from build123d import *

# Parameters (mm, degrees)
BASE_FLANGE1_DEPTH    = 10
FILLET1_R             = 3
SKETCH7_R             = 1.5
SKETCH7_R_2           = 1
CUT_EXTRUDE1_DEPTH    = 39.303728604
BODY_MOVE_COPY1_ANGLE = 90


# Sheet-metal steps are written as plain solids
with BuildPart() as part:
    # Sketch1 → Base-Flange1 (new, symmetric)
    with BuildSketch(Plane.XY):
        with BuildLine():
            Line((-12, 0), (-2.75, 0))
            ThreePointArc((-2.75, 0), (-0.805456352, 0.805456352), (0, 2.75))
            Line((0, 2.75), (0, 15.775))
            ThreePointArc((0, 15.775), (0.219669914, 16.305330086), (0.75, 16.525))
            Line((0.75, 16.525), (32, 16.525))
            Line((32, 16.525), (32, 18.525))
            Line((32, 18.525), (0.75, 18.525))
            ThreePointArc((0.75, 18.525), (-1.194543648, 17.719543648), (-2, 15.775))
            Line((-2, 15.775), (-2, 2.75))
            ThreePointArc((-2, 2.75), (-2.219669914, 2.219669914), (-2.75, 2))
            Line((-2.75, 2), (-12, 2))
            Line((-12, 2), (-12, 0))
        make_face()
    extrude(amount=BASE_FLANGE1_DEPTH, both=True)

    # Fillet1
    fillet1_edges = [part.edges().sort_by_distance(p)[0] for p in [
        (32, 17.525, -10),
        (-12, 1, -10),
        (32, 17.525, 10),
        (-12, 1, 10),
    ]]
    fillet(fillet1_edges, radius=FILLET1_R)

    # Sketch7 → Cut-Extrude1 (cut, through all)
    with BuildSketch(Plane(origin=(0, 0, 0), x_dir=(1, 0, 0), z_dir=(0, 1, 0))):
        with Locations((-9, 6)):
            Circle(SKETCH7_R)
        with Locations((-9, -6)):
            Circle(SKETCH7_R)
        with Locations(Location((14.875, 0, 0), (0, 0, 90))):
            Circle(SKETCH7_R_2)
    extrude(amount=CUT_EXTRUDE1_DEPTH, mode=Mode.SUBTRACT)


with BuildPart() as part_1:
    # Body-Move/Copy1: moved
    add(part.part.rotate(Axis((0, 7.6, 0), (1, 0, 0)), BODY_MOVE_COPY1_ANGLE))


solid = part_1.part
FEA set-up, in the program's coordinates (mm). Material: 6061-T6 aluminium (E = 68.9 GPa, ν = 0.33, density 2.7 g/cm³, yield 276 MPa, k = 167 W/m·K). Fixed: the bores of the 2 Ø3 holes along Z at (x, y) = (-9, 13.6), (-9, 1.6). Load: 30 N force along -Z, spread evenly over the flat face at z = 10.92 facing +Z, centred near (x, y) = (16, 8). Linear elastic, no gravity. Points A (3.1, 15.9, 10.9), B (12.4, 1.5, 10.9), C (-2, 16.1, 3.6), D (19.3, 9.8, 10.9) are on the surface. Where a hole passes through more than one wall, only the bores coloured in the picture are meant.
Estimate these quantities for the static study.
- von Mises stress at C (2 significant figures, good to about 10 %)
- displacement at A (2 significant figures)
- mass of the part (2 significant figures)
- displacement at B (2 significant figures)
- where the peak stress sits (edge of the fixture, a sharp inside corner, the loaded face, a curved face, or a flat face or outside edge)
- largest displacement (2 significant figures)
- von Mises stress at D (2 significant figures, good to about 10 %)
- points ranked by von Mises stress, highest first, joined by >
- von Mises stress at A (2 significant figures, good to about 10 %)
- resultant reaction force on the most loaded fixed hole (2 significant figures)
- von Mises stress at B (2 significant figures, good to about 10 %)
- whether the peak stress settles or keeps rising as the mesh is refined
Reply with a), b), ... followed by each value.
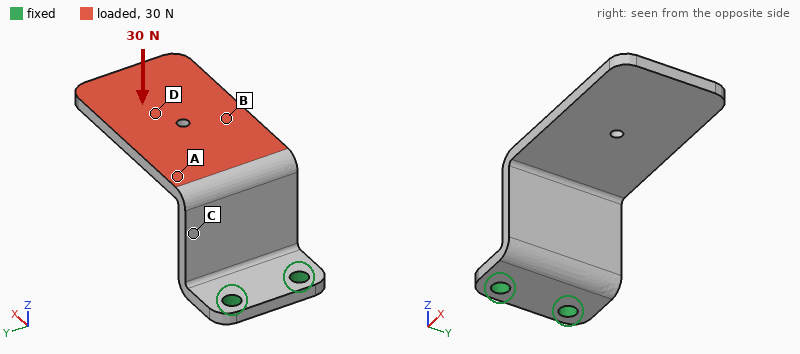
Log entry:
a) 38 MPa
b) 0.18 mm
c) 6.2 g
d) 0.28 mm
e) edge of the fixture
f) 0.61 mm
g) 5.6 MPa
h) C > A > B > D
i) 29 MPa
j) 17 N
k) 14 MPa
l) keeps rising
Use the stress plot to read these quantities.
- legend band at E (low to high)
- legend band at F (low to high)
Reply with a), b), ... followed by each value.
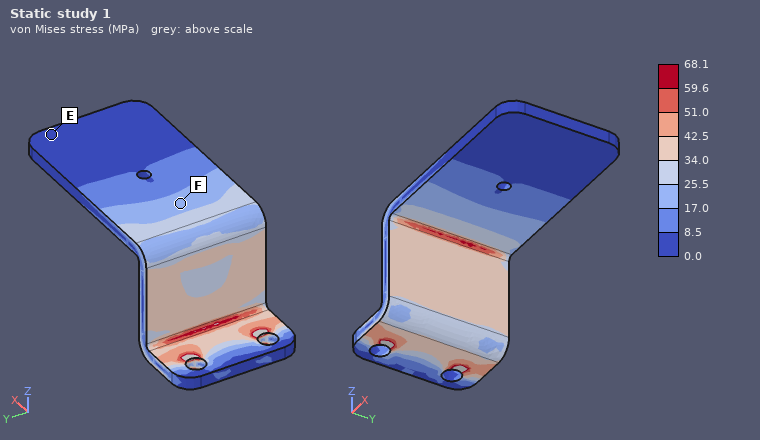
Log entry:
a) 0.0 to 8.5 MPa
b) 17.0 to 25.5 MPa
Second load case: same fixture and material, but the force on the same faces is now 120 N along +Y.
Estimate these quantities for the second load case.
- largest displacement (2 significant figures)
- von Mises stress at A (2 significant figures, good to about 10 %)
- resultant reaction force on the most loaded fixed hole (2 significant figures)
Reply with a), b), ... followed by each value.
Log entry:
a) 0.56 mm
b) 39 MPa
c) 270 N
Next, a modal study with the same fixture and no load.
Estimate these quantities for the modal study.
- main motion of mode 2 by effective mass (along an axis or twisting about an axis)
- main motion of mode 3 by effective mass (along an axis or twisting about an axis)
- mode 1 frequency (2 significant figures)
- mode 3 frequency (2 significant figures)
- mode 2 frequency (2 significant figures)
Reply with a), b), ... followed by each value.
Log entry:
a) along Y
b) along X
c) 700 Hz
d) 2400 Hz
e) 1500 Hz
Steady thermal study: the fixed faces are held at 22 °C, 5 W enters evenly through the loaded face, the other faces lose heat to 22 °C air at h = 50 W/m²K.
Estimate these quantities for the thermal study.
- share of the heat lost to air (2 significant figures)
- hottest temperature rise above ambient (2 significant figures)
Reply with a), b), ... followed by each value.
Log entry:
a) 24 %
b) 24 K
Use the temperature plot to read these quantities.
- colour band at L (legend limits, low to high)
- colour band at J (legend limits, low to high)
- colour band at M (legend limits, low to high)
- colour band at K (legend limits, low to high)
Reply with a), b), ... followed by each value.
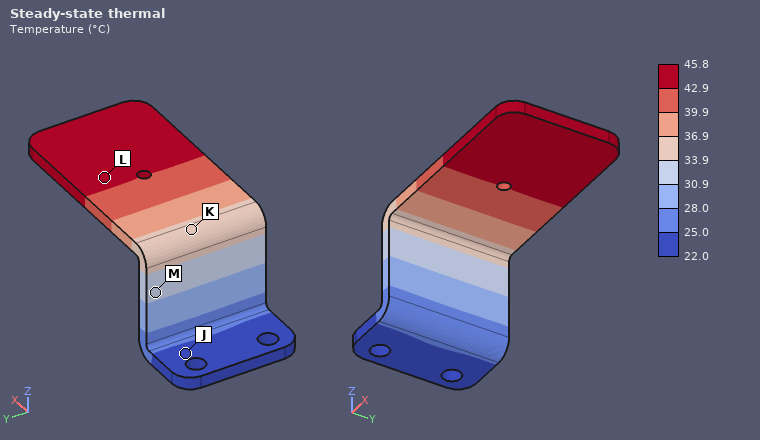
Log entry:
a) 42.9 to 45.8 °C
b) 22.0 to 25.0 °C
c) 30.9 to 33.9 °C
d) 33.9 to 36.9 °C
